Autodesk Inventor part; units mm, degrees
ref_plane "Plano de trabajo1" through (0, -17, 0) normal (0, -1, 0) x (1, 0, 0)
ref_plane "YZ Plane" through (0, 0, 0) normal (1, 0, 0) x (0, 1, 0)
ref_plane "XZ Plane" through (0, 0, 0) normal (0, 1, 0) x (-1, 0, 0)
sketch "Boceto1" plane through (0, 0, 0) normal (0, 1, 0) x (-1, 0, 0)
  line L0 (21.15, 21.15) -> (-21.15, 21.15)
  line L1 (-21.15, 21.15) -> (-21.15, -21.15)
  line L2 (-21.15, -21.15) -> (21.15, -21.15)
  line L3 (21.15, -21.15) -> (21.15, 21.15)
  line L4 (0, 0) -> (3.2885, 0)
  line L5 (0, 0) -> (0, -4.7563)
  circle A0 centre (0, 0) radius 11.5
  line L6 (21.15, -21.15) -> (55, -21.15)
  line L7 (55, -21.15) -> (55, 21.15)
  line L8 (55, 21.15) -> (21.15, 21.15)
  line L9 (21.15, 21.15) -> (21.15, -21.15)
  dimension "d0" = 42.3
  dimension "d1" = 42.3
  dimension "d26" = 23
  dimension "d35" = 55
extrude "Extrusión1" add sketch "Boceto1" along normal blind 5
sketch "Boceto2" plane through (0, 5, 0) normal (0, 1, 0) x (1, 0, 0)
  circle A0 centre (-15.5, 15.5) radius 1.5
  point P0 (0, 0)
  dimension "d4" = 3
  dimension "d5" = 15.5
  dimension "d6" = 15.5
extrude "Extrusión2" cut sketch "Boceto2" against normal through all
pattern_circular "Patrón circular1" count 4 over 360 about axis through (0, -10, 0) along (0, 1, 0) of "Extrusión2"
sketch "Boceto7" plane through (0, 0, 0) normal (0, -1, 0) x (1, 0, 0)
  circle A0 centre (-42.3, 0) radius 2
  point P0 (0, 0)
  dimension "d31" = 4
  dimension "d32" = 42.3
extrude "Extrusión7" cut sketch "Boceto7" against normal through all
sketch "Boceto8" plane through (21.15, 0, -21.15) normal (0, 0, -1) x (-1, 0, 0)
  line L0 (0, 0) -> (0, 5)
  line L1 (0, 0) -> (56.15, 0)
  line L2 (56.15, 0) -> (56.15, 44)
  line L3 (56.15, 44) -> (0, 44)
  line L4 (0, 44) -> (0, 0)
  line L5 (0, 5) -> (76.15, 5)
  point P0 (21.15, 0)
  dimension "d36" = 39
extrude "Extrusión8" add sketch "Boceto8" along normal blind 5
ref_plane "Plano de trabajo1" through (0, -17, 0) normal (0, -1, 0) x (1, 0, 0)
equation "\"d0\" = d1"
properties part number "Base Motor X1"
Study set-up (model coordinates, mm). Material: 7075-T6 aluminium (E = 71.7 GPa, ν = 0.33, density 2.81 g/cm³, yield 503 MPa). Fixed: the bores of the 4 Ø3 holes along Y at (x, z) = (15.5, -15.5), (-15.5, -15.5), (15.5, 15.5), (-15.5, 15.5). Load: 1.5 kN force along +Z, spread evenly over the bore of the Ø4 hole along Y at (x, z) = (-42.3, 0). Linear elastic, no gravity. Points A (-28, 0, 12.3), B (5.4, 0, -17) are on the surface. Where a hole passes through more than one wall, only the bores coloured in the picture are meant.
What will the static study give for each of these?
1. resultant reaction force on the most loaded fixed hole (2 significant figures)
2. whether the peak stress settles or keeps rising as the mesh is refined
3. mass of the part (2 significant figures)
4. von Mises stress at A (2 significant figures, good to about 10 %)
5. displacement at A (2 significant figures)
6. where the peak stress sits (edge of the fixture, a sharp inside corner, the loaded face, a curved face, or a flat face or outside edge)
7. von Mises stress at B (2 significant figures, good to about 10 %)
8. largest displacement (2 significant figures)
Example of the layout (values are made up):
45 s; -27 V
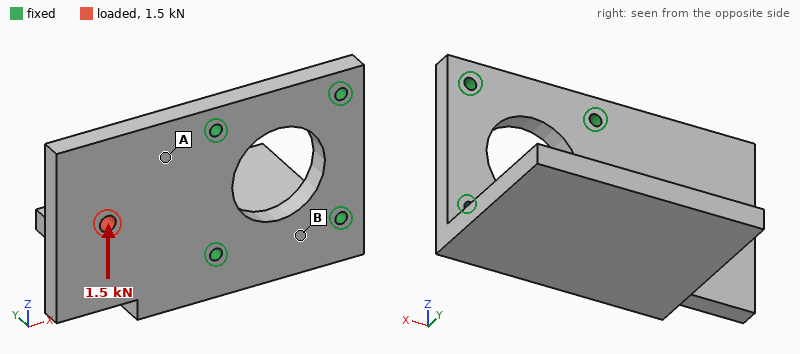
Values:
1.3 kN; keeps rising; 74 g; 14 MPa; 5.5 µm; edge of the fixture; 4.0 MPa; 17 µm
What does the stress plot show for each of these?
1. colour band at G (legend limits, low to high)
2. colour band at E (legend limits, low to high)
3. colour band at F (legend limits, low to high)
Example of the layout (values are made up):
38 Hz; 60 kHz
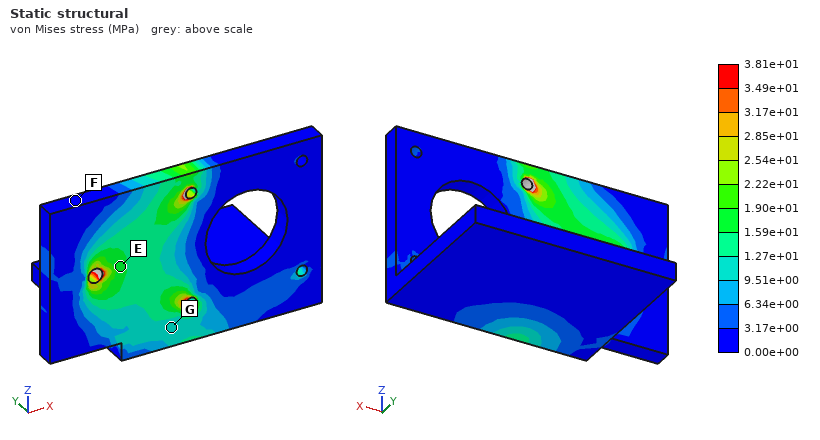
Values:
9.51e+00 to 1.27e+01 MPa; 1.59e+01 to 1.90e+01 MPa; 0.00e+00 to 3.17e+00 MPa
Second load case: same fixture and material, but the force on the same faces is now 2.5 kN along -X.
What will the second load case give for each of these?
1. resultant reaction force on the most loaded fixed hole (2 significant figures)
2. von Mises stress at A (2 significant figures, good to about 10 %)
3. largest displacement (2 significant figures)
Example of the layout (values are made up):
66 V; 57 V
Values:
1.2 kN; 16 MPa; 11 µm
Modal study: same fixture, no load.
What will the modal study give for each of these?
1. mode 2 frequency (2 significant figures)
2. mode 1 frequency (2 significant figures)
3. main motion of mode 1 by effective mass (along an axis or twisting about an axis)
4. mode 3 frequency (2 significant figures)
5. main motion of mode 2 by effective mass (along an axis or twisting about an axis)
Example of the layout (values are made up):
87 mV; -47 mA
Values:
3000 Hz; 1700 Hz; along Z; 3900 Hz; along Y
